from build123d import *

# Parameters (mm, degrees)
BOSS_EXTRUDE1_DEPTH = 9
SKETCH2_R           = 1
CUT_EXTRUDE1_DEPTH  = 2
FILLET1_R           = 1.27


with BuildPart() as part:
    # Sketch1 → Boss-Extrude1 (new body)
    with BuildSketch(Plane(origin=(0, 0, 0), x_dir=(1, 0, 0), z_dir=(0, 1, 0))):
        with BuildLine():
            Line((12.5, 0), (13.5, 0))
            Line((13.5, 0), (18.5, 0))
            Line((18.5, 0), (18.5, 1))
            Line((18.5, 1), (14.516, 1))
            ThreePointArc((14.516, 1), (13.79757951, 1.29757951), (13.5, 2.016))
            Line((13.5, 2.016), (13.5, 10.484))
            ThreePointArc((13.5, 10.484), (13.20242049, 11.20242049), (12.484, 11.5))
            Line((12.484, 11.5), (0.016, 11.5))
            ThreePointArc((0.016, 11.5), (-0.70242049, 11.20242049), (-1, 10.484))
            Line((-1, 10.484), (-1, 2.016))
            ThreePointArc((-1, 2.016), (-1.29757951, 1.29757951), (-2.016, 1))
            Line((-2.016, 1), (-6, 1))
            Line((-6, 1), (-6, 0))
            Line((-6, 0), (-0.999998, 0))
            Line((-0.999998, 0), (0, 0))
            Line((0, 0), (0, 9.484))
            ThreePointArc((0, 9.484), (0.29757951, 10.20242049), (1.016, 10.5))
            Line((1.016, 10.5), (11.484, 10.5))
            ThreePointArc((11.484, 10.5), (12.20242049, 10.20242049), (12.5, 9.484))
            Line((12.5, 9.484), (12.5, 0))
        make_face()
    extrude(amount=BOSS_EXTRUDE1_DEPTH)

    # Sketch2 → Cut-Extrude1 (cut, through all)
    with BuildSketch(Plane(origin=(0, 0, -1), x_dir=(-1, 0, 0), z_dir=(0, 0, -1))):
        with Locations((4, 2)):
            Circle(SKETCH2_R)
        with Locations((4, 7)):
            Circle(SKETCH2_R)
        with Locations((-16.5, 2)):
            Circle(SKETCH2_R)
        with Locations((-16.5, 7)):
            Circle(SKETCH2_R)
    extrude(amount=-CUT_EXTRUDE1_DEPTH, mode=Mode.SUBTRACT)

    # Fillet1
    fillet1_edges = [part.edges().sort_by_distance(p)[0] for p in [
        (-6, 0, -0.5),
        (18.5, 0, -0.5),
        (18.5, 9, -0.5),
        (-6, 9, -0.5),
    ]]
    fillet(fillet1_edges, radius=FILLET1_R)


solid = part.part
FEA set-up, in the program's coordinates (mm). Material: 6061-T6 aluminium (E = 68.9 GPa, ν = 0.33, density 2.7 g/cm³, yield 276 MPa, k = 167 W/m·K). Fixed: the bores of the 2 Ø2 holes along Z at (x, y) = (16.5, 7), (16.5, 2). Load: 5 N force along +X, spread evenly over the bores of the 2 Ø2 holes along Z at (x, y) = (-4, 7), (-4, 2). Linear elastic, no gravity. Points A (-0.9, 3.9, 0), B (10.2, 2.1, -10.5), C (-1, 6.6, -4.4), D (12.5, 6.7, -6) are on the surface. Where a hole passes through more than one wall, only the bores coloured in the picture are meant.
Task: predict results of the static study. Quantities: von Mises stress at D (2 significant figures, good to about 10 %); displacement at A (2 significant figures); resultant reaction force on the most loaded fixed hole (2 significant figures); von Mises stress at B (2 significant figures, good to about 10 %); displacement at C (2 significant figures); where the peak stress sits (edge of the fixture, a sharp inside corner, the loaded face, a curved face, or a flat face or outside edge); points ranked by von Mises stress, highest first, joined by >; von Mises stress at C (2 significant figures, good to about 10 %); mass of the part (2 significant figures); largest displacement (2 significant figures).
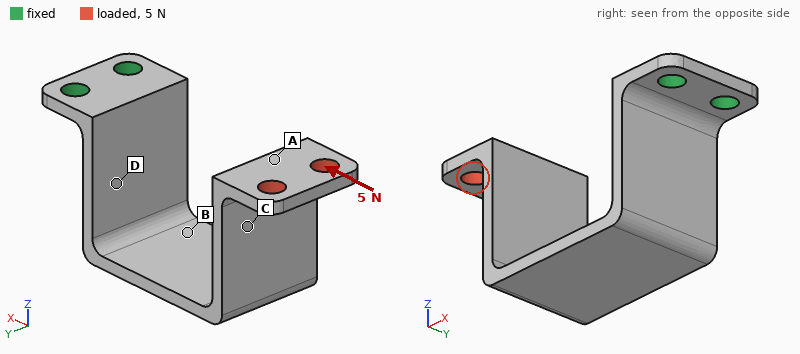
17 MPa
0.24 mm
2.5 N
34 MPa
0.18 mm
a curved face
B > D > C > A
12 MPa
1.1 g
0.32 mm
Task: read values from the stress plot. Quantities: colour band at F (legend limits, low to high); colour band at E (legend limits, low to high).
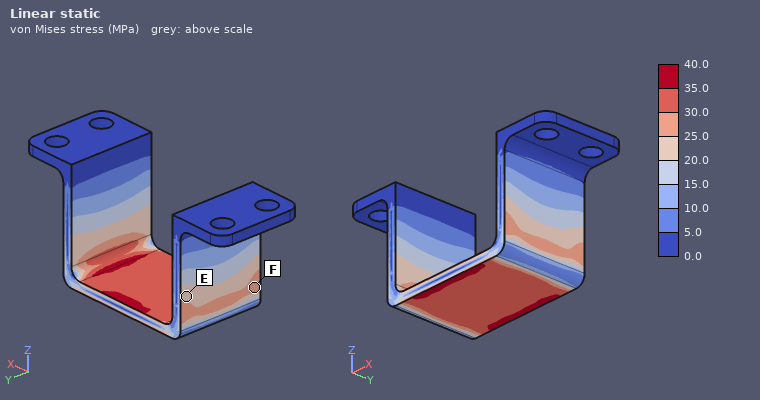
25.0 to 30.0 MPa
20.0 to 25.0 MPa
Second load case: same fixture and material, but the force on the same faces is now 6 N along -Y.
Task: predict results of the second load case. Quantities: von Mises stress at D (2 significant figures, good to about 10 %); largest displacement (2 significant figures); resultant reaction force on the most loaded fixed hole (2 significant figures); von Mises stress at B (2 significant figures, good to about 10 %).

57 MPa
0.33 mm
20 N
42 MPa
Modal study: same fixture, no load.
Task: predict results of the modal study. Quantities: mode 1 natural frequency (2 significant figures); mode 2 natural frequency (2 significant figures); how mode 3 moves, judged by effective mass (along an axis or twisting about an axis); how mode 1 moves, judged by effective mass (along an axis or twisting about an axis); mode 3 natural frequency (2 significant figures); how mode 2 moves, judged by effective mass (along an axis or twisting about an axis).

870 Hz
1400 Hz
along X
along Z
2000 Hz
along Y
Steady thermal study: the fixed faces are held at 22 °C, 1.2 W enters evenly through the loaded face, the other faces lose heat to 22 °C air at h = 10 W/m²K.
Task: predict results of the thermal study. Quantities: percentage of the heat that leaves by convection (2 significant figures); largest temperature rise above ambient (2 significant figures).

9.8 %
29 K
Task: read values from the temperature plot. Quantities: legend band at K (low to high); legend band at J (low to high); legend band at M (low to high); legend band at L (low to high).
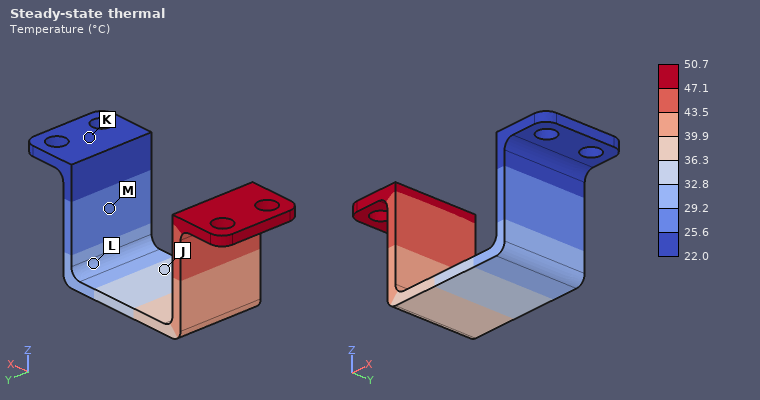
22.0 to 25.6 °C
32.8 to 36.3 °C
25.6 to 29.2 °C
29.2 to 32.8 °C
